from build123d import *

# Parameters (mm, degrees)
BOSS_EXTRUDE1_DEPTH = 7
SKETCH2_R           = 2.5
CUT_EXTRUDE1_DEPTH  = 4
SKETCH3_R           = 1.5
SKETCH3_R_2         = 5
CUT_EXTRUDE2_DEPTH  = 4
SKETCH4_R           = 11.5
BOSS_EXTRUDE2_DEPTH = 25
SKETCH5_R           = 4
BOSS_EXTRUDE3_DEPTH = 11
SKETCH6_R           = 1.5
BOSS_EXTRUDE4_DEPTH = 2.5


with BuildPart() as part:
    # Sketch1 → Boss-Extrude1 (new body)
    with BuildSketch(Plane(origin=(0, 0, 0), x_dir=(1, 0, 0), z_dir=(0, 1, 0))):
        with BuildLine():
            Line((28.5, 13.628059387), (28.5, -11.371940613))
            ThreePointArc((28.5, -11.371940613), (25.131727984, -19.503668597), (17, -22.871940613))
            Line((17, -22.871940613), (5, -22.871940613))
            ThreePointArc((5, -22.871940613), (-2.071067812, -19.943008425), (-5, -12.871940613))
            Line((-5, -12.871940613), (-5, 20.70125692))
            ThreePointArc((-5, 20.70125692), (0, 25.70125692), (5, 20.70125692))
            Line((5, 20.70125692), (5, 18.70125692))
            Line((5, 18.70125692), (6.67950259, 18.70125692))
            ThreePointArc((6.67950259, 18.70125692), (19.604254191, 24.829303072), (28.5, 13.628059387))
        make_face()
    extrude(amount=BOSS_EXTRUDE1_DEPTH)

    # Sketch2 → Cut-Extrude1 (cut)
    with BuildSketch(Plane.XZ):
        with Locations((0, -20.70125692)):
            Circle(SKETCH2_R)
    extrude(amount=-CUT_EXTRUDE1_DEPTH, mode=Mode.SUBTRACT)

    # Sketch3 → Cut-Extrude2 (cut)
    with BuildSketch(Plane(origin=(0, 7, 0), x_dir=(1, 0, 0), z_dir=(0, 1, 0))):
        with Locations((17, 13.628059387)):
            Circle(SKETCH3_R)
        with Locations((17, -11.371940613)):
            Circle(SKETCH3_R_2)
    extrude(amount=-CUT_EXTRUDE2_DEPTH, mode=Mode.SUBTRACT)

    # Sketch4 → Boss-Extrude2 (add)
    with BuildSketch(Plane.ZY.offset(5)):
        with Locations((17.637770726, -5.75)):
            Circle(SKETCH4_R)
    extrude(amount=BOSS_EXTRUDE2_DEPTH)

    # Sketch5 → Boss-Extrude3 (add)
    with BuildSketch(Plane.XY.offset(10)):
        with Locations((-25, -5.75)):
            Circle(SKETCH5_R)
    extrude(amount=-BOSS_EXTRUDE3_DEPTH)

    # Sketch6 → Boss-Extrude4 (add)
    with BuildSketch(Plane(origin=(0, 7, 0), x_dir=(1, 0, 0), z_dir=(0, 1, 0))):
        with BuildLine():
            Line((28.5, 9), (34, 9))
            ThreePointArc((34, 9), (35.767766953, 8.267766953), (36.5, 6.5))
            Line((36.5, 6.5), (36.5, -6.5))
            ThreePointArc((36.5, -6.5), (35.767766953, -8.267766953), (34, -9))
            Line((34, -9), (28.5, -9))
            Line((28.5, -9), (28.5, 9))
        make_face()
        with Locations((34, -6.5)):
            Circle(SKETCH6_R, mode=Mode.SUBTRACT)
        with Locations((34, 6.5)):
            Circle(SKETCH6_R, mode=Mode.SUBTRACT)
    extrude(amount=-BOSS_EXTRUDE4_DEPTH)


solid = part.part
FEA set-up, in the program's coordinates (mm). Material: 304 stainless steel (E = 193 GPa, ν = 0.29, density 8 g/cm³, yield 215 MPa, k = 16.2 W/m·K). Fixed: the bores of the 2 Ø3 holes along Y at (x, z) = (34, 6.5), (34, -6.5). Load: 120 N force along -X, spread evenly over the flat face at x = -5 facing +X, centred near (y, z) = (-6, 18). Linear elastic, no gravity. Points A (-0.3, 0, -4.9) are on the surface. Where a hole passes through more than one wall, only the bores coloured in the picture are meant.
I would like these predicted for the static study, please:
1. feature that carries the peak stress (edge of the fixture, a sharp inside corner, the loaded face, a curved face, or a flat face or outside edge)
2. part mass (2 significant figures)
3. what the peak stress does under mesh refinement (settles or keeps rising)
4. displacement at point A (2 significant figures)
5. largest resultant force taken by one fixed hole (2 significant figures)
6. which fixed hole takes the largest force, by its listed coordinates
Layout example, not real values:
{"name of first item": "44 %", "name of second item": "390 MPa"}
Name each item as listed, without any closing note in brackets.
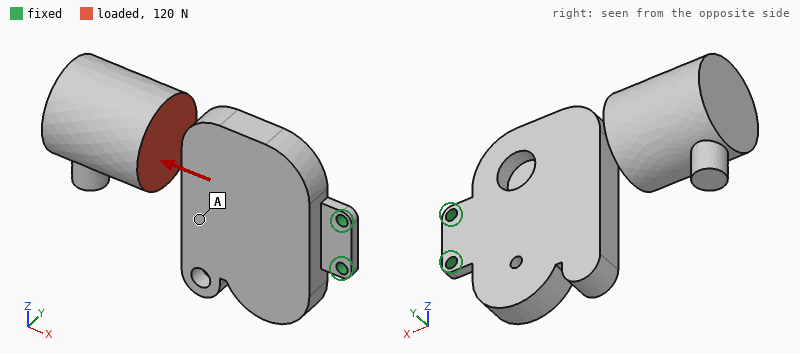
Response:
{"feature that carries the peak stress": "edge of the fixture", "part mass": "170 g", "what the peak stress does under mesh refinement": "keeps rising", "displacement at point A": "0.060 mm", "largest resultant force taken by one fixed hole": "220 N", "which fixed hole takes the largest force, by its listed coordinates": "(34, 6.5)"}
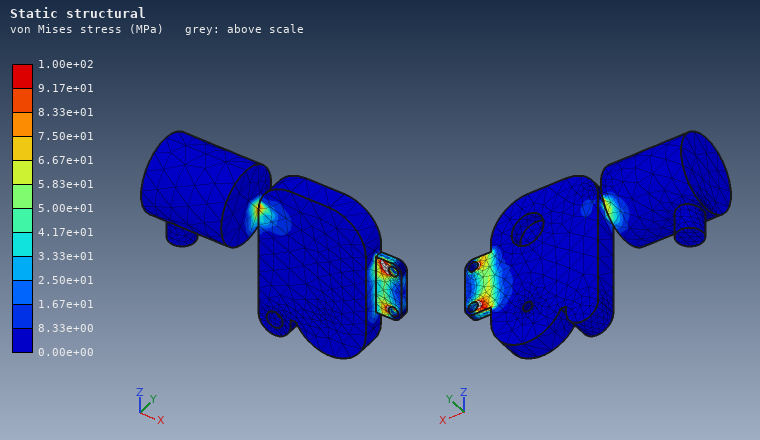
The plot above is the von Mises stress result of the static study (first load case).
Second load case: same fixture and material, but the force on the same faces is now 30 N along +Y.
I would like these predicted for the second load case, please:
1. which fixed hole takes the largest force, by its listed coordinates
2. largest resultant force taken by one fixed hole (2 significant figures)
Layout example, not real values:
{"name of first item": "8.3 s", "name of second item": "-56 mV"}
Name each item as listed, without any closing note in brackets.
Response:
{"which fixed hole takes the largest force, by its listed coordinates": "(34, 6.5)", "largest resultant force taken by one fixed hole": "54 N"}
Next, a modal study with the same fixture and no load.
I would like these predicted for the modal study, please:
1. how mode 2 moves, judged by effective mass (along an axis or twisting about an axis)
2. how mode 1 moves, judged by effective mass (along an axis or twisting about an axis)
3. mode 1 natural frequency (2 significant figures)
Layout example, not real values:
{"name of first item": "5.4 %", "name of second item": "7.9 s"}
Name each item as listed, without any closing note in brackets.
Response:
{"how mode 2 moves, judged by effective mass": "along Z", "how mode 1 moves, judged by effective mass": "along Y", "mode 1 natural frequency": "260 Hz"}
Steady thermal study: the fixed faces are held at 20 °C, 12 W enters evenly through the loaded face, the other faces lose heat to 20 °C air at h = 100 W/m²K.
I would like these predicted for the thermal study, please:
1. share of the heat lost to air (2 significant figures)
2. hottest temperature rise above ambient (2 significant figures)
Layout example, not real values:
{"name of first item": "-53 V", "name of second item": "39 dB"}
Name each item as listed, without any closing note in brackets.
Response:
{"share of the heat lost to air": "98 %", "hottest temperature rise above ambient": "59 K"}
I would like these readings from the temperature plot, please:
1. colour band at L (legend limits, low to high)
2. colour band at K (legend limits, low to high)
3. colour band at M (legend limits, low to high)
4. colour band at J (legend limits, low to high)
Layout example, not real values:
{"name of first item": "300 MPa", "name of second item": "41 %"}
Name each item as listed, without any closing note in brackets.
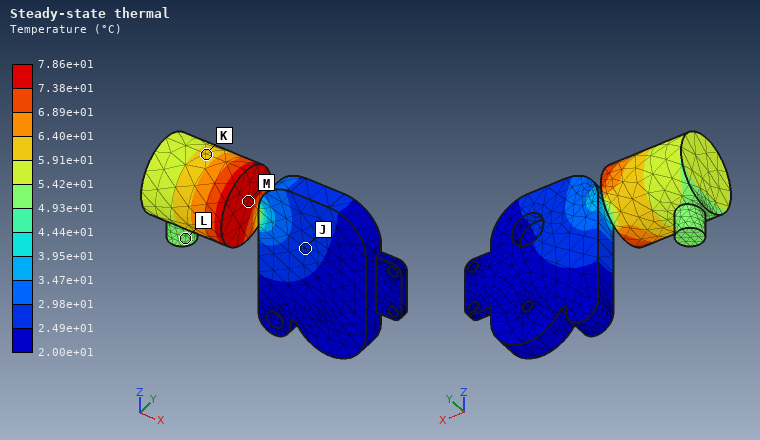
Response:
{"colour band at L": "4.93e+01 to 5.42e+01 °C", "colour band at K": "5.91e+01 to 6.40e+01 °C", "colour band at M": "7.38e+01 to 7.86e+01 °C", "colour band at J": "2.49e+01 to 2.98e+01 °C"}
